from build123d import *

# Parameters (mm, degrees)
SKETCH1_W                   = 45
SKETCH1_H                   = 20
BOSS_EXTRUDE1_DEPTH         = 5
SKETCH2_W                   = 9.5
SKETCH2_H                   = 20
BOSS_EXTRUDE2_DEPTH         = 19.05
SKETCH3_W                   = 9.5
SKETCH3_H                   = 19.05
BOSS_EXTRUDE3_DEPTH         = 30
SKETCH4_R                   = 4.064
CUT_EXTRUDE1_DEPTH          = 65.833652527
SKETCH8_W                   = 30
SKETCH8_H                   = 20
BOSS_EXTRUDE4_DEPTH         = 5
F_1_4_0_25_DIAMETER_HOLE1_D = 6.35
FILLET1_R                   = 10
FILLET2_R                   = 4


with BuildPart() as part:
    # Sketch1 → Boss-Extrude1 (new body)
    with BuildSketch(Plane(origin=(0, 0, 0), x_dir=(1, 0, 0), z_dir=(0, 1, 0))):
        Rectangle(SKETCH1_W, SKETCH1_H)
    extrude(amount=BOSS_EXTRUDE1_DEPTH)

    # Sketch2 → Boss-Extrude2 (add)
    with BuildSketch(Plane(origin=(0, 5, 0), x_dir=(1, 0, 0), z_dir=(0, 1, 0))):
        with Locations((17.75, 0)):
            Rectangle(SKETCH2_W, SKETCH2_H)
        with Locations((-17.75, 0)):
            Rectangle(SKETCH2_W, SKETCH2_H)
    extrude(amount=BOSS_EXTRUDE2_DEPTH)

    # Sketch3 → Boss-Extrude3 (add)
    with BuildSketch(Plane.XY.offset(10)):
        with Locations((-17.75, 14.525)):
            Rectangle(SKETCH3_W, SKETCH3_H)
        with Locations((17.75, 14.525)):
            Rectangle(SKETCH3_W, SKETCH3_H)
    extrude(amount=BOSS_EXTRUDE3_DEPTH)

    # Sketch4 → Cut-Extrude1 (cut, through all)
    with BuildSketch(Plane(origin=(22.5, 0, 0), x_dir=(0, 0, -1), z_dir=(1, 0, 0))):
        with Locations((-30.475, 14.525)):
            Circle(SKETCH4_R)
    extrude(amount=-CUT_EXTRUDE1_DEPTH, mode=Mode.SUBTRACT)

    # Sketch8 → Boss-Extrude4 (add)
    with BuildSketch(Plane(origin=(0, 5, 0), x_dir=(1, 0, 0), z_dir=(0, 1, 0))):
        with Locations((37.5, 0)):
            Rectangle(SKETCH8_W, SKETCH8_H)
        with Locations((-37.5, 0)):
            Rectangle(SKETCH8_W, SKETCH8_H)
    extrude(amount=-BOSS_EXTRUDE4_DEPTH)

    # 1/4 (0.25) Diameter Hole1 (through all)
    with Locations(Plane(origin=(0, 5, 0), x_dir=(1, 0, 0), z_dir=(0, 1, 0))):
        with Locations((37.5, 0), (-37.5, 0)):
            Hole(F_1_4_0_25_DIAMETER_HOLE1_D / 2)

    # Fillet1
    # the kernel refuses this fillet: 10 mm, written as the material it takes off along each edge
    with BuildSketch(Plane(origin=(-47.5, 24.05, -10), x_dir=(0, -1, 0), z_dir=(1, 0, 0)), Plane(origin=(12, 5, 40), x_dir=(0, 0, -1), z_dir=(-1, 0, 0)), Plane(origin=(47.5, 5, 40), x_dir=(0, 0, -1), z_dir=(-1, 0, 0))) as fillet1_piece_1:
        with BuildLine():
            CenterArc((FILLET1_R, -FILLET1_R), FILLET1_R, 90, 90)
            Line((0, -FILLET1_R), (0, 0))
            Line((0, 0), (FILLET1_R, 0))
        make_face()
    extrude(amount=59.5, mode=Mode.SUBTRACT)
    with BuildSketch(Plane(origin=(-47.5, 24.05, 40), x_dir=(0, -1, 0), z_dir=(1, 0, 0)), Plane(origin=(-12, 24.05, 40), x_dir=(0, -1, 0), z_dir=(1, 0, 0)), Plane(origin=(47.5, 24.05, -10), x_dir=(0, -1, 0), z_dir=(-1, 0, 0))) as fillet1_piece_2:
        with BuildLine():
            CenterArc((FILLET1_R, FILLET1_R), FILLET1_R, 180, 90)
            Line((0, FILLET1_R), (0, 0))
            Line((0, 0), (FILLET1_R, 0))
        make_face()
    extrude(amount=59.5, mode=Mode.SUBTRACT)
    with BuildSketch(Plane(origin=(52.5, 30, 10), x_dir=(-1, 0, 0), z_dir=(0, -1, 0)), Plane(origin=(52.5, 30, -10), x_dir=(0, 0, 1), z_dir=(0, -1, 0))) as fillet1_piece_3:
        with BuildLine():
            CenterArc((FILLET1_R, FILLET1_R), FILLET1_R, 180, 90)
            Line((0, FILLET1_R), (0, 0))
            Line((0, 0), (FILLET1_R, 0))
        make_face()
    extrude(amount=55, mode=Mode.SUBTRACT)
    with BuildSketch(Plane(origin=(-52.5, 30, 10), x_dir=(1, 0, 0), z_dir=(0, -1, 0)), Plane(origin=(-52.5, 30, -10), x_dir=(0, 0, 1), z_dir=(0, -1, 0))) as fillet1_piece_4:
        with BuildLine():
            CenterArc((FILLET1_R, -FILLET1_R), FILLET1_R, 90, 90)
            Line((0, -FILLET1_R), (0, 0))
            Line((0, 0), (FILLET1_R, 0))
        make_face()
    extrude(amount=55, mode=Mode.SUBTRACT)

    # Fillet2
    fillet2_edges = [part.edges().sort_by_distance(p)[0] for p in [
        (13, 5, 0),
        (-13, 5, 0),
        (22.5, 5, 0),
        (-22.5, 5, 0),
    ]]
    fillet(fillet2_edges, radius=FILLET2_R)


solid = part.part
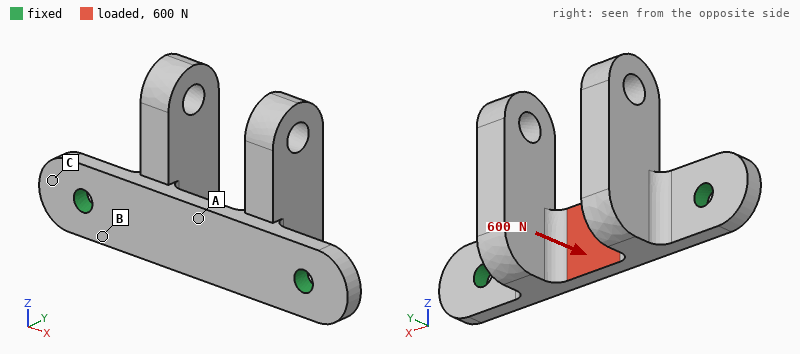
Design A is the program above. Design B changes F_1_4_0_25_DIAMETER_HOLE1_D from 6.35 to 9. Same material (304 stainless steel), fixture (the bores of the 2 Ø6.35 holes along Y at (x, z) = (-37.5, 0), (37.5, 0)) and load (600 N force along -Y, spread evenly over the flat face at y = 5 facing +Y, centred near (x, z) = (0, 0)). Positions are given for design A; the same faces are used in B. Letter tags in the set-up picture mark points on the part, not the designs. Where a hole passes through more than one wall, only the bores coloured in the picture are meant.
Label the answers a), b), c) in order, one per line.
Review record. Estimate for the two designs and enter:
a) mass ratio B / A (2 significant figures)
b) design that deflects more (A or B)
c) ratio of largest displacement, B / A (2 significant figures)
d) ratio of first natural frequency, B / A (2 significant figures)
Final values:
a) 0.99
b) A
c) 0.88
d) 1.1
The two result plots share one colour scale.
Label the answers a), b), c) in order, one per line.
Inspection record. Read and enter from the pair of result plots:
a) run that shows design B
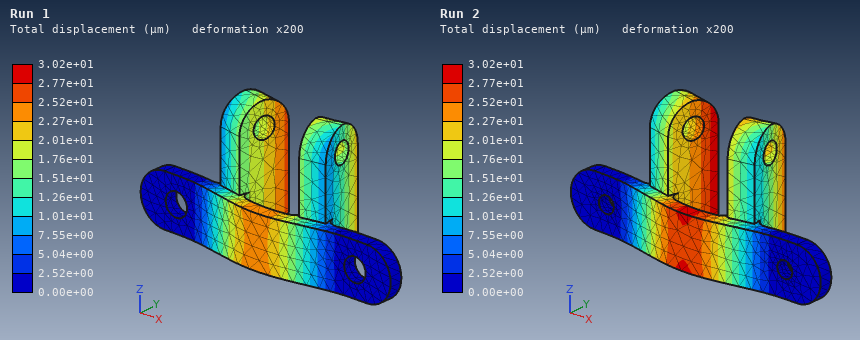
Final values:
a) Run 1
